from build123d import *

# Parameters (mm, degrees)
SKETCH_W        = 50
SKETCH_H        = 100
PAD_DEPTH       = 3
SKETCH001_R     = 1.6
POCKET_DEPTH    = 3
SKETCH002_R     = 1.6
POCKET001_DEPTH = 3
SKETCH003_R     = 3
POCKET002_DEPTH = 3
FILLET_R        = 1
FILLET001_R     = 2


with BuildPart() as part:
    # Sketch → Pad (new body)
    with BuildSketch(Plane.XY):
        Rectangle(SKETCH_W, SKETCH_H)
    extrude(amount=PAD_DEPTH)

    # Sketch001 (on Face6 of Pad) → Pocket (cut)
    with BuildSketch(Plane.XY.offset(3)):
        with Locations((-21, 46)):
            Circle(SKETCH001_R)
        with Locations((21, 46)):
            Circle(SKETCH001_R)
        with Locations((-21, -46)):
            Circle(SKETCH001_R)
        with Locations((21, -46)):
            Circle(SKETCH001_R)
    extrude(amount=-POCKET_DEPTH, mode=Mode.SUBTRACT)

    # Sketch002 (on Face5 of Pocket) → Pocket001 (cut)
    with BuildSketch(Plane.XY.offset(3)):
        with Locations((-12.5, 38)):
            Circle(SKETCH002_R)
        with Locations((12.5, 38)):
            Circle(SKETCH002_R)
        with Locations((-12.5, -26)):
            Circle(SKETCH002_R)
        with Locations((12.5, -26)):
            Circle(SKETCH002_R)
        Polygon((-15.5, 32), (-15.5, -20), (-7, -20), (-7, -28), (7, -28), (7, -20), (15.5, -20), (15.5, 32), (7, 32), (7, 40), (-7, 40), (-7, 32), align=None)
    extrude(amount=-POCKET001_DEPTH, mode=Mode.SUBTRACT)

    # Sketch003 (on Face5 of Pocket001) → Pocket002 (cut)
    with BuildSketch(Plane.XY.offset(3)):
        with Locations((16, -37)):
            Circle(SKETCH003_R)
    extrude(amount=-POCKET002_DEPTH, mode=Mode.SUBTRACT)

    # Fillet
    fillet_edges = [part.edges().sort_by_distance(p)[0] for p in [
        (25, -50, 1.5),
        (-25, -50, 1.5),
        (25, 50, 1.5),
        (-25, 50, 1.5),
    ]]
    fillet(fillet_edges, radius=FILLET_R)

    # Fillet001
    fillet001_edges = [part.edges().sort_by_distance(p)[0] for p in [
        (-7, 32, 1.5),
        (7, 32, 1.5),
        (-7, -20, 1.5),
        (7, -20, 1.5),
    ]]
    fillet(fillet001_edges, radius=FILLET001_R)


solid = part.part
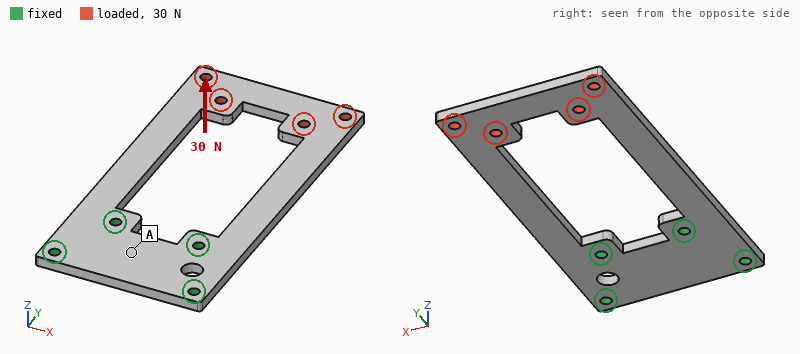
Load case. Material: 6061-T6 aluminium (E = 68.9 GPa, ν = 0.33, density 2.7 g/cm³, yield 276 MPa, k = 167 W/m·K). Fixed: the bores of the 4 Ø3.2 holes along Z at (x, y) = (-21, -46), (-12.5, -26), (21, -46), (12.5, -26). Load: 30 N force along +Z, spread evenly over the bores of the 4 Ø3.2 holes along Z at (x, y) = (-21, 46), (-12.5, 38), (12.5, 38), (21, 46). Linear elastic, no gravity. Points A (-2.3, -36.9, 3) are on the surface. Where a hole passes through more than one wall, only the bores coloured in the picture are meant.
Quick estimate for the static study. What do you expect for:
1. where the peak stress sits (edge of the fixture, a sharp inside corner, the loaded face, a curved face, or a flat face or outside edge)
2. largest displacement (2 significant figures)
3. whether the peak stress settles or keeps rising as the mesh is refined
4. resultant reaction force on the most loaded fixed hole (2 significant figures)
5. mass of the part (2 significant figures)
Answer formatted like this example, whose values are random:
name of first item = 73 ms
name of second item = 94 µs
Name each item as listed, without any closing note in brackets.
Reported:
where the peak stress sits = edge of the fixture
largest displacement = 1.3 mm
whether the peak stress settles or keeps rising as the mesh is refined = keeps rising
resultant reaction force on the most loaded fixed hole = 38 N
mass of the part = 25 g
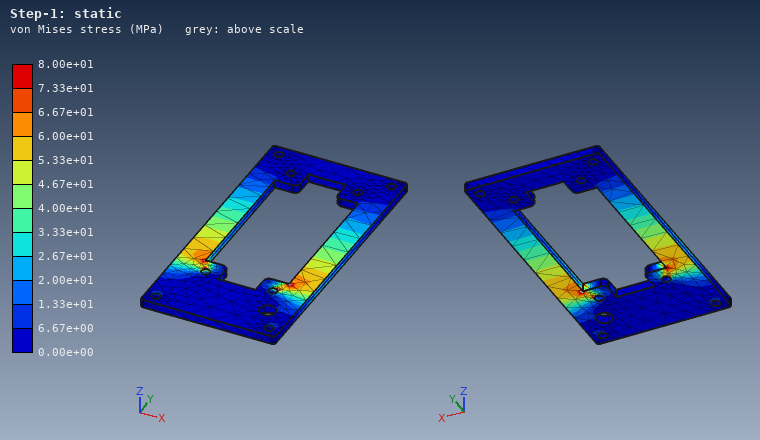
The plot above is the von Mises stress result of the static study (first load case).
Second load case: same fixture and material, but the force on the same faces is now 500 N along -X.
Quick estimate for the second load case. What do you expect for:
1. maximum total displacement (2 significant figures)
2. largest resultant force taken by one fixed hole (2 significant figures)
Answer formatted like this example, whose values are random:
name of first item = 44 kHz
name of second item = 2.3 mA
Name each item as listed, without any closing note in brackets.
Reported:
maximum total displacement = 0.47 mm
largest resultant force taken by one fixed hole = 630 N
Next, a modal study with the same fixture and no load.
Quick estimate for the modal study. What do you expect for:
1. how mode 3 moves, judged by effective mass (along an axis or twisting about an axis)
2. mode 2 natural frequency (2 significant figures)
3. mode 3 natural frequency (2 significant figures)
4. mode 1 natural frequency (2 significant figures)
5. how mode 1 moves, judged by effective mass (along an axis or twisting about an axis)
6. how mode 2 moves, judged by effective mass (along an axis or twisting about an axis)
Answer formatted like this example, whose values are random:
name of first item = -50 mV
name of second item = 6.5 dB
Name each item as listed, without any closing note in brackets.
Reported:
how mode 3 moves, judged by effective mass = along X
mode 2 natural frequency = 950 Hz
mode 3 natural frequency = 1800 Hz
mode 1 natural frequency = 310 Hz
how mode 1 moves, judged by effective mass = along Z
how mode 2 moves, judged by effective mass = twisting about Y
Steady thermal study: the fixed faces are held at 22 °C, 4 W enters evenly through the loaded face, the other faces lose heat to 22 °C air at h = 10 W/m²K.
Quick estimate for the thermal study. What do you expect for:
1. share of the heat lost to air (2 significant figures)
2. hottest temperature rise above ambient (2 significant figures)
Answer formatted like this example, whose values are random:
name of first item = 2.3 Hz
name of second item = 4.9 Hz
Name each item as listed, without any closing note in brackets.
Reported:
share of the heat lost to air = 19 %
hottest temperature rise above ambient = 24 K
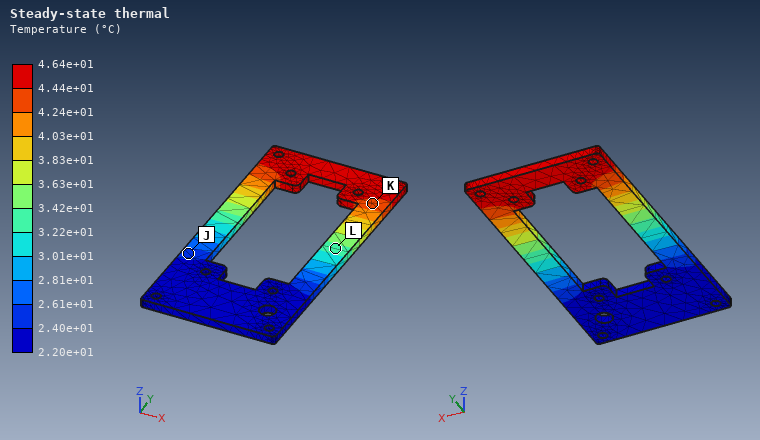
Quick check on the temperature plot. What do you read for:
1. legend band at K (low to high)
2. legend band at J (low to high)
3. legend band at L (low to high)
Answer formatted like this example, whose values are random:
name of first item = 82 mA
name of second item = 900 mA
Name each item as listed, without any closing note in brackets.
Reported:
legend band at K = 4.24e+01 to 4.44e+01 °C
legend band at J = 2.40e+01 to 2.61e+01 °C
legend band at L = 3.22e+01 to 3.42e+01 °C
